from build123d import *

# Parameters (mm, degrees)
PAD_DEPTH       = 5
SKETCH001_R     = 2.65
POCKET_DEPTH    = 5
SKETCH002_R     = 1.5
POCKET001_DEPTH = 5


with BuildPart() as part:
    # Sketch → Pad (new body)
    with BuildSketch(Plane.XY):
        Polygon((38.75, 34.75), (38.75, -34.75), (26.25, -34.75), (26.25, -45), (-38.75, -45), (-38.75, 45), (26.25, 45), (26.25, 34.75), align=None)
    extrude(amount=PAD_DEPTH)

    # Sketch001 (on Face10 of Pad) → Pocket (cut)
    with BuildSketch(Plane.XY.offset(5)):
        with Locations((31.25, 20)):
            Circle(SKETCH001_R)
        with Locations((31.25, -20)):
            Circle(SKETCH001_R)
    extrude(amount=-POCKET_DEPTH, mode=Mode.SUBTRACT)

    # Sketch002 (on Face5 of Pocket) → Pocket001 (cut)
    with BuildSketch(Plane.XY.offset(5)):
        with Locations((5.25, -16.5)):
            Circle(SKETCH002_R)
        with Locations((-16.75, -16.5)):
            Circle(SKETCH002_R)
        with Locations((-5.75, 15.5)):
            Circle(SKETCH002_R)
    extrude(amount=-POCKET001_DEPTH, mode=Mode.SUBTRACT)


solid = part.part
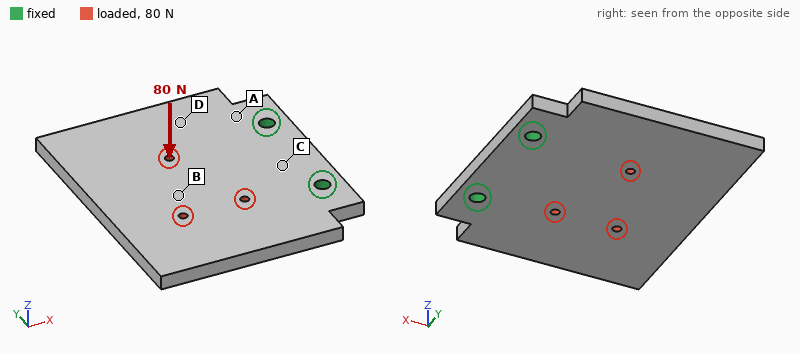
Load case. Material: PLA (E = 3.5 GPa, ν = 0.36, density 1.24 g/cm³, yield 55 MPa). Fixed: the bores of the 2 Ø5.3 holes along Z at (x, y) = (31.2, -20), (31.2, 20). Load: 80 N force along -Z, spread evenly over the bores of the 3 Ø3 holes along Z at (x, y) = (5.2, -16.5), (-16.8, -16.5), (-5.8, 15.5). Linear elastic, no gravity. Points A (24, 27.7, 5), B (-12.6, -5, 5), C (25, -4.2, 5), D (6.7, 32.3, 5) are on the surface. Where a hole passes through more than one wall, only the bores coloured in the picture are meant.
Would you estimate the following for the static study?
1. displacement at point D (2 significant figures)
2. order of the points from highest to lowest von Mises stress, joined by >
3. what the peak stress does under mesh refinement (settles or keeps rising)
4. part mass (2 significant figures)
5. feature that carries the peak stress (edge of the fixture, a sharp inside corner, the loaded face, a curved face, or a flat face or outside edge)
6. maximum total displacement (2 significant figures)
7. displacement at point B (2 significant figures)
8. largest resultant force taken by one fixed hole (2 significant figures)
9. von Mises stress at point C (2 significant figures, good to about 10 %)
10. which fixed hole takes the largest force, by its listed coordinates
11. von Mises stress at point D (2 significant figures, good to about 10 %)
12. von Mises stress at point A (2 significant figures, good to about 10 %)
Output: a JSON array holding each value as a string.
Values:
["0.24 mm", "A > C > D > B", "keeps rising", "41 g", "edge of the fixture", "1.3 mm", "0.71 mm", "50 N", "5.0 MPa", "(31.2, -20)", "2.8 MPa", "6.6 MPa"]
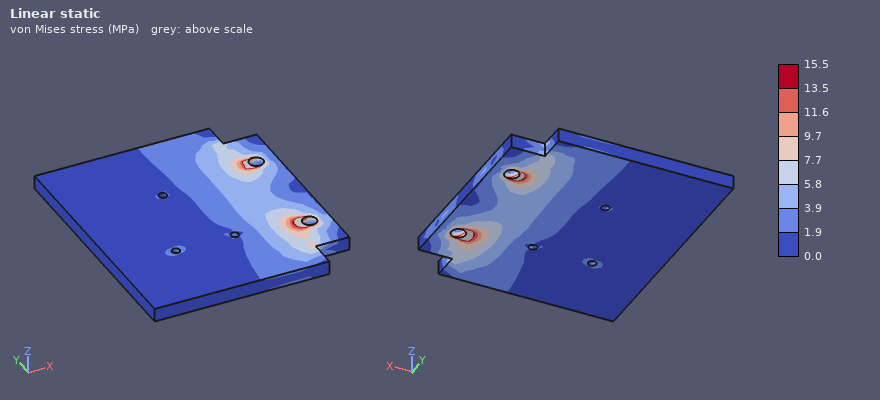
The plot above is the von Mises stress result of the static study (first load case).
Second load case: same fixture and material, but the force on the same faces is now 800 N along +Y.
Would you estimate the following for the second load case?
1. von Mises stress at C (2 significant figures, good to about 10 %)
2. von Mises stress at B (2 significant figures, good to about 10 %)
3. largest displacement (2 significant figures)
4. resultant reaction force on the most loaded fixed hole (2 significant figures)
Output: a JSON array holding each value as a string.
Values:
["5.2 MPa", "2.5 MPa", "0.25 mm", "780 N"]
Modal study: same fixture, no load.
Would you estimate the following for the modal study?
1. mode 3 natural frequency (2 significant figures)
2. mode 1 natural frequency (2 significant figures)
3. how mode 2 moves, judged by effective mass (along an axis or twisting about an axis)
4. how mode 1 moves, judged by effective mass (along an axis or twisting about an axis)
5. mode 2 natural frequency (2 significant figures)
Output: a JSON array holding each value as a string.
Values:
["1200 Hz", "250 Hz", "twisting about X", "along Z", "480 Hz"]
